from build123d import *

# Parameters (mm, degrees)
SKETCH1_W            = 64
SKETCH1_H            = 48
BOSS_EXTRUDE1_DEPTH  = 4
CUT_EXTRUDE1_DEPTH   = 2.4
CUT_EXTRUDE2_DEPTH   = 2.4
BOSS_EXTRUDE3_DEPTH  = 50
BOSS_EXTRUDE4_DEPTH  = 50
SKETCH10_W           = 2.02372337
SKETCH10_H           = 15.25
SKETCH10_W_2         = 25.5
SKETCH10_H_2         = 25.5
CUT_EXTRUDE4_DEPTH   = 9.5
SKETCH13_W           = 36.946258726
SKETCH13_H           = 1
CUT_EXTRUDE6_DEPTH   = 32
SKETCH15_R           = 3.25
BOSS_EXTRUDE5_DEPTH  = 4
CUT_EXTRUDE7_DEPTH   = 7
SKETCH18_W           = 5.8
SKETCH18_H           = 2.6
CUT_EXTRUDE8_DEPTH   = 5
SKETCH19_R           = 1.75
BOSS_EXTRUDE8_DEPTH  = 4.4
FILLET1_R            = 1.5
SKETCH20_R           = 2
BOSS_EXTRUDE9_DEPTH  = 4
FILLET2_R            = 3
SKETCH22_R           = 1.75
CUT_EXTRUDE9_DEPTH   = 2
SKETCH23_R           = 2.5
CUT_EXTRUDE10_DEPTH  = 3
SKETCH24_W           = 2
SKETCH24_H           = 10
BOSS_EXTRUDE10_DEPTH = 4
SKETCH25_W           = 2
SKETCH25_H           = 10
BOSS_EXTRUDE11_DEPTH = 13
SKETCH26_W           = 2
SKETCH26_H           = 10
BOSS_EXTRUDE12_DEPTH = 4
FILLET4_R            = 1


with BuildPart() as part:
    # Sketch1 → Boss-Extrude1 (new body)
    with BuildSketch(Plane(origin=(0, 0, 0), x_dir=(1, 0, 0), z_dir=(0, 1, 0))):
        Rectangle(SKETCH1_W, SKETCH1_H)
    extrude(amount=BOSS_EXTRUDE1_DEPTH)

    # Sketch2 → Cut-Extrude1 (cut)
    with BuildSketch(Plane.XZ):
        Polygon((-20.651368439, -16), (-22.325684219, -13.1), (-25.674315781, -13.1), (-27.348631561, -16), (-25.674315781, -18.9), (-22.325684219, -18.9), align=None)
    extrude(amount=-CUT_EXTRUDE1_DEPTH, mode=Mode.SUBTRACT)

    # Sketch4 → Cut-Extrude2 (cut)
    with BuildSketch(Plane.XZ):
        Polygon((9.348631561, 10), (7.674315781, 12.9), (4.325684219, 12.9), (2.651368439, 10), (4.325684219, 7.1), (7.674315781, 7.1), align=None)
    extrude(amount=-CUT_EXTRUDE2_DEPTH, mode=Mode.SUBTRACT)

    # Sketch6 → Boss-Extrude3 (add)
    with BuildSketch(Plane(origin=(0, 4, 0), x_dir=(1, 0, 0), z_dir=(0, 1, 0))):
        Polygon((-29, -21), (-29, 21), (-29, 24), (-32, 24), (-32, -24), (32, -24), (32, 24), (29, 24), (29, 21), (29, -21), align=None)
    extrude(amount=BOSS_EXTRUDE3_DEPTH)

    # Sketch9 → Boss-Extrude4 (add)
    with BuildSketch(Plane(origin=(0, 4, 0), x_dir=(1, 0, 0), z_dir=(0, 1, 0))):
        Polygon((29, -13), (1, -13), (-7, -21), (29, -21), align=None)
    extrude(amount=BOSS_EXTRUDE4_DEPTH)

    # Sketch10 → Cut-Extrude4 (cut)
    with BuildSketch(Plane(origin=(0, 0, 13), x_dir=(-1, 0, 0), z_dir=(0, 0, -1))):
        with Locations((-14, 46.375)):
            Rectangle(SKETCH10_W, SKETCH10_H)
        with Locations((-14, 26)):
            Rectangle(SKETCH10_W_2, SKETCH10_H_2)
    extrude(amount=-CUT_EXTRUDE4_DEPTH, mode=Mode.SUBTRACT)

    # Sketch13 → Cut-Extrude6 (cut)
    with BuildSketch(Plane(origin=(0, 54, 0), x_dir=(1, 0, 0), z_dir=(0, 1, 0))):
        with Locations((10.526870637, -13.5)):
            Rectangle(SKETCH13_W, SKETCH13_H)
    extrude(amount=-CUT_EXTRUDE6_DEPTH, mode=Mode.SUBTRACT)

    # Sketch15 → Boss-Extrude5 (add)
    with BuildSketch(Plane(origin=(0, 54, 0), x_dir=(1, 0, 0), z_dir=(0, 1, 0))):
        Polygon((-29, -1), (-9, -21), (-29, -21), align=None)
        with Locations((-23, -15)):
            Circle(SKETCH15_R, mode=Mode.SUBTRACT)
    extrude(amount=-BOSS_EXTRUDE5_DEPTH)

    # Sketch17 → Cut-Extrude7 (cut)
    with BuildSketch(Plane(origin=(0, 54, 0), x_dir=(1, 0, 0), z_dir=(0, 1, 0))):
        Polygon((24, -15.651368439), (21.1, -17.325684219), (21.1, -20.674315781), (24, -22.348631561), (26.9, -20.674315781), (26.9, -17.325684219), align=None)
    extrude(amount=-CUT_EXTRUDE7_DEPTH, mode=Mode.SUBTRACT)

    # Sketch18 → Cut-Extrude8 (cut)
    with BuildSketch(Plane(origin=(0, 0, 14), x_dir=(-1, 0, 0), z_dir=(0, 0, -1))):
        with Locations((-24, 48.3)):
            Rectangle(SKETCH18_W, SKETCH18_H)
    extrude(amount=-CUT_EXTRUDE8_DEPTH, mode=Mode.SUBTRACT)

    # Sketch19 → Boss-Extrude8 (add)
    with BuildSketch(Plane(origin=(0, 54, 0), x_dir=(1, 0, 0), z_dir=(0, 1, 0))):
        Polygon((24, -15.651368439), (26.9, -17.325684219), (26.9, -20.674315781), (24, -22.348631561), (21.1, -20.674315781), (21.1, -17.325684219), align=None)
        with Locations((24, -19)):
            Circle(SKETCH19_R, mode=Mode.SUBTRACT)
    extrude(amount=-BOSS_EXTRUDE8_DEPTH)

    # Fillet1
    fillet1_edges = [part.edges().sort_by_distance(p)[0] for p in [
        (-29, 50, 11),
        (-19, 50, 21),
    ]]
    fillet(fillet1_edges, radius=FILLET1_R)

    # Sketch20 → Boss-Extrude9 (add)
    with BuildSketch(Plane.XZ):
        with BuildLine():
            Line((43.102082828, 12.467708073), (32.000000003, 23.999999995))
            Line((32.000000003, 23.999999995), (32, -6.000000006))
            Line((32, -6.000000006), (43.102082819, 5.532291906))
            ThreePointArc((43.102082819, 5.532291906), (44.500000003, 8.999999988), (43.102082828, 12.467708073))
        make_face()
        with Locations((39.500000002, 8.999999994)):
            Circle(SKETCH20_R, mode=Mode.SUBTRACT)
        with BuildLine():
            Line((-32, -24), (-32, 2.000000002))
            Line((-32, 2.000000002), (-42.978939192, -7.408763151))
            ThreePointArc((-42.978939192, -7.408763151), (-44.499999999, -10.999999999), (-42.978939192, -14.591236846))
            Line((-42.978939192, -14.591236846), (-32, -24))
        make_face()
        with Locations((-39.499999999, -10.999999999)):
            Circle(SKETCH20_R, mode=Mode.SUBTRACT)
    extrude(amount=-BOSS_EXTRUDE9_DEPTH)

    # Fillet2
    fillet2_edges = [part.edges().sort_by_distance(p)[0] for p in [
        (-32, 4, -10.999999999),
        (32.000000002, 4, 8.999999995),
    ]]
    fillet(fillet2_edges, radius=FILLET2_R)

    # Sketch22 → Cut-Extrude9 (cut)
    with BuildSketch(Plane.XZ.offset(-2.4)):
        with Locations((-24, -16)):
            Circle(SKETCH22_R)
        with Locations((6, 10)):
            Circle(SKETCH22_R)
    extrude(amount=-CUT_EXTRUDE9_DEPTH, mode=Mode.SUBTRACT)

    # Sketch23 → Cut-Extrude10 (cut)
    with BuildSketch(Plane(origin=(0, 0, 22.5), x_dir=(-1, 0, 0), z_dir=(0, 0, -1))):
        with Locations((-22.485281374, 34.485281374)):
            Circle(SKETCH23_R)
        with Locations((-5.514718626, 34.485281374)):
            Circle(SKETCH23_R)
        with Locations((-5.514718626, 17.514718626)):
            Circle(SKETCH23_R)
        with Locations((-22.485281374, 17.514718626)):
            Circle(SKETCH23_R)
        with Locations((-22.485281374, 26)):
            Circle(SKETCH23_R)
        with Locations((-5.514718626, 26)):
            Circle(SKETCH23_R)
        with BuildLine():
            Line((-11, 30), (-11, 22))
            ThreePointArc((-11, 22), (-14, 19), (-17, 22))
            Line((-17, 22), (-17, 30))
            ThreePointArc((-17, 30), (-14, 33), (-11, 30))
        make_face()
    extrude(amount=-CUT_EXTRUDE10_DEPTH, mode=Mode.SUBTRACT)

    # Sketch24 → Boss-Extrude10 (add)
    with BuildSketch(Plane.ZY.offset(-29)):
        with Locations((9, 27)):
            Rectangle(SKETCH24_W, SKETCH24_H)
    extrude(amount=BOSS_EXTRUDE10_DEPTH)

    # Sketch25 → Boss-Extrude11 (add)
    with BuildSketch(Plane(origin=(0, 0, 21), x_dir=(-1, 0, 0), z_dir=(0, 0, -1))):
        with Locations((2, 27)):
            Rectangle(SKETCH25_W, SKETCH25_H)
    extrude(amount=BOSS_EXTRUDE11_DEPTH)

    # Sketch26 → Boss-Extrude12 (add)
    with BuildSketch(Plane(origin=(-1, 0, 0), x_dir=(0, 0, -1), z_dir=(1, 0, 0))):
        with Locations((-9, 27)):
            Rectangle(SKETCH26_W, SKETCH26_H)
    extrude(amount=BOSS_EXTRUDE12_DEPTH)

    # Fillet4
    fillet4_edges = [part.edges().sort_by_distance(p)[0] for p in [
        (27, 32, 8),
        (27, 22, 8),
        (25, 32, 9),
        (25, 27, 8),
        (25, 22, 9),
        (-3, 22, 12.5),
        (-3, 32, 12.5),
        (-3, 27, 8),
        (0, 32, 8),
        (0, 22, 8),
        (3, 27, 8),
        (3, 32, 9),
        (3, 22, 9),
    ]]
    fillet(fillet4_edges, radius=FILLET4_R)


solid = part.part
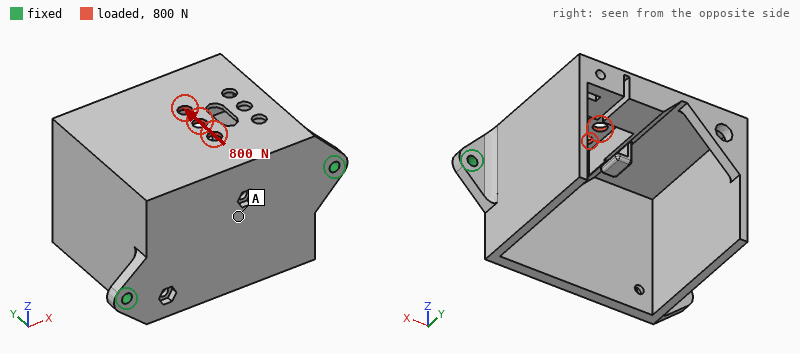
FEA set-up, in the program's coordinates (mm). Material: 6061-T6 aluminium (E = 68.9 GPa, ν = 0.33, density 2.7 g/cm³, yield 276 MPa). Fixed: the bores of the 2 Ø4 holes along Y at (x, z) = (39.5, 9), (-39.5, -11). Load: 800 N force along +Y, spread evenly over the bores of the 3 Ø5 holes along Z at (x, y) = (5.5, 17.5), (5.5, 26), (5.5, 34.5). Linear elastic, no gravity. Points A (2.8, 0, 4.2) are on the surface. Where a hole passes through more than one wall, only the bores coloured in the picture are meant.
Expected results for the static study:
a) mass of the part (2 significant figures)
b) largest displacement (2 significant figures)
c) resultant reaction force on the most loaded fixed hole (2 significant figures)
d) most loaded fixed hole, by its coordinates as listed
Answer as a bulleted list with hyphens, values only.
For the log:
- 120 g
- 0.41 mm
- 510 N
- (39.5, 9)
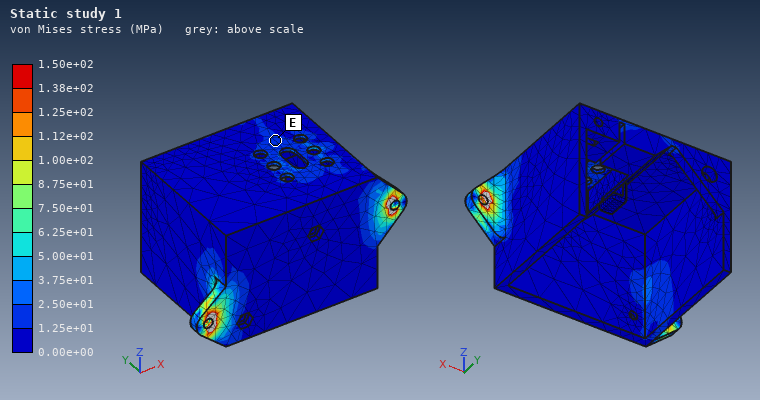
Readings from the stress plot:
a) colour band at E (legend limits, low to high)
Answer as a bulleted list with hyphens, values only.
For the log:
- 1.25e+01 to 2.50e+01 MPa
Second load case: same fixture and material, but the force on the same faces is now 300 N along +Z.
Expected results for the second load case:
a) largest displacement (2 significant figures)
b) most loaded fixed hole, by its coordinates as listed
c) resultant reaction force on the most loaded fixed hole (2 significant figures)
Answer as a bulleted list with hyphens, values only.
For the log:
- 0.17 mm
- (39.5, 9)
- 170 N
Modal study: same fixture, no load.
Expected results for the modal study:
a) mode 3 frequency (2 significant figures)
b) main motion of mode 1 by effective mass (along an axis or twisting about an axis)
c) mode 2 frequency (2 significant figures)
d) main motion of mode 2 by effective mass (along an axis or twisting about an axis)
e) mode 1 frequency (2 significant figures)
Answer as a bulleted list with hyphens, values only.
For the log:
- 1900 Hz
- along Z
- 1400 Hz
- along X
- 790 Hz
